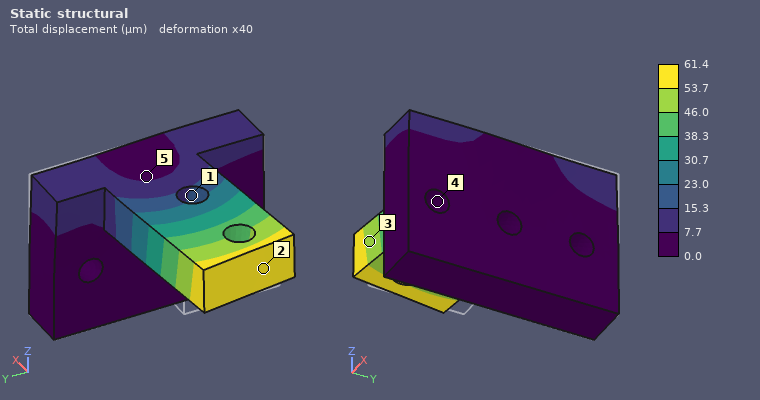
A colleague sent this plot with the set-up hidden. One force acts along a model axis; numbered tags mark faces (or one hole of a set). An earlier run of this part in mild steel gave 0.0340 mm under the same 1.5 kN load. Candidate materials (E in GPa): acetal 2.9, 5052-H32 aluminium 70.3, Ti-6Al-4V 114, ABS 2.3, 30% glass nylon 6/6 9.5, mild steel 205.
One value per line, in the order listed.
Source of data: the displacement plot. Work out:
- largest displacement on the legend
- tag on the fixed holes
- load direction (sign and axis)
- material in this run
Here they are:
61.4 µm
4
-Y
Ti-6Al-4V
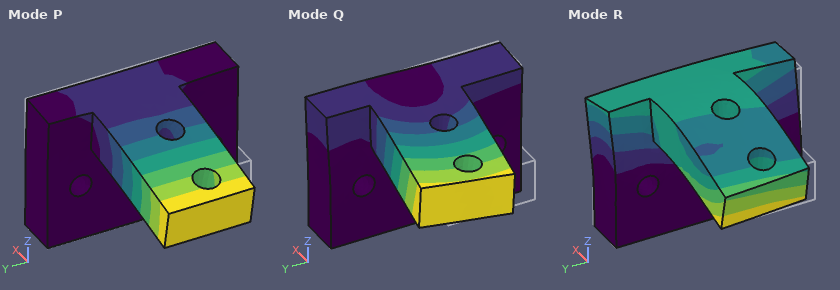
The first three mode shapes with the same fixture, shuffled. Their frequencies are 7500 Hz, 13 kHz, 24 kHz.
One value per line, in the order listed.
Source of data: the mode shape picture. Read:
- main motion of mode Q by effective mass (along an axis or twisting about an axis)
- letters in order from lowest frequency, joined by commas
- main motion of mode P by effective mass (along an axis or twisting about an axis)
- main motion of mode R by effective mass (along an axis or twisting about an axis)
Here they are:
along Y
P, Q, R
along Z
along X
